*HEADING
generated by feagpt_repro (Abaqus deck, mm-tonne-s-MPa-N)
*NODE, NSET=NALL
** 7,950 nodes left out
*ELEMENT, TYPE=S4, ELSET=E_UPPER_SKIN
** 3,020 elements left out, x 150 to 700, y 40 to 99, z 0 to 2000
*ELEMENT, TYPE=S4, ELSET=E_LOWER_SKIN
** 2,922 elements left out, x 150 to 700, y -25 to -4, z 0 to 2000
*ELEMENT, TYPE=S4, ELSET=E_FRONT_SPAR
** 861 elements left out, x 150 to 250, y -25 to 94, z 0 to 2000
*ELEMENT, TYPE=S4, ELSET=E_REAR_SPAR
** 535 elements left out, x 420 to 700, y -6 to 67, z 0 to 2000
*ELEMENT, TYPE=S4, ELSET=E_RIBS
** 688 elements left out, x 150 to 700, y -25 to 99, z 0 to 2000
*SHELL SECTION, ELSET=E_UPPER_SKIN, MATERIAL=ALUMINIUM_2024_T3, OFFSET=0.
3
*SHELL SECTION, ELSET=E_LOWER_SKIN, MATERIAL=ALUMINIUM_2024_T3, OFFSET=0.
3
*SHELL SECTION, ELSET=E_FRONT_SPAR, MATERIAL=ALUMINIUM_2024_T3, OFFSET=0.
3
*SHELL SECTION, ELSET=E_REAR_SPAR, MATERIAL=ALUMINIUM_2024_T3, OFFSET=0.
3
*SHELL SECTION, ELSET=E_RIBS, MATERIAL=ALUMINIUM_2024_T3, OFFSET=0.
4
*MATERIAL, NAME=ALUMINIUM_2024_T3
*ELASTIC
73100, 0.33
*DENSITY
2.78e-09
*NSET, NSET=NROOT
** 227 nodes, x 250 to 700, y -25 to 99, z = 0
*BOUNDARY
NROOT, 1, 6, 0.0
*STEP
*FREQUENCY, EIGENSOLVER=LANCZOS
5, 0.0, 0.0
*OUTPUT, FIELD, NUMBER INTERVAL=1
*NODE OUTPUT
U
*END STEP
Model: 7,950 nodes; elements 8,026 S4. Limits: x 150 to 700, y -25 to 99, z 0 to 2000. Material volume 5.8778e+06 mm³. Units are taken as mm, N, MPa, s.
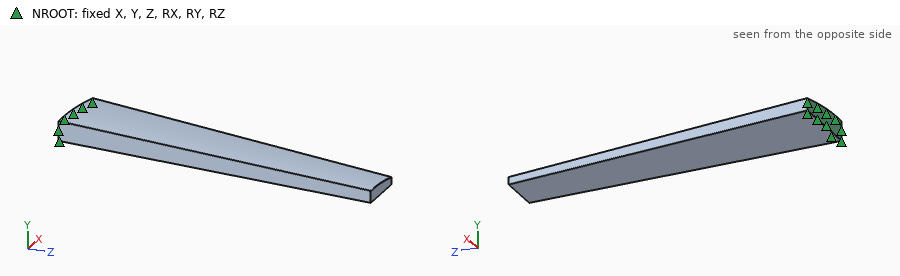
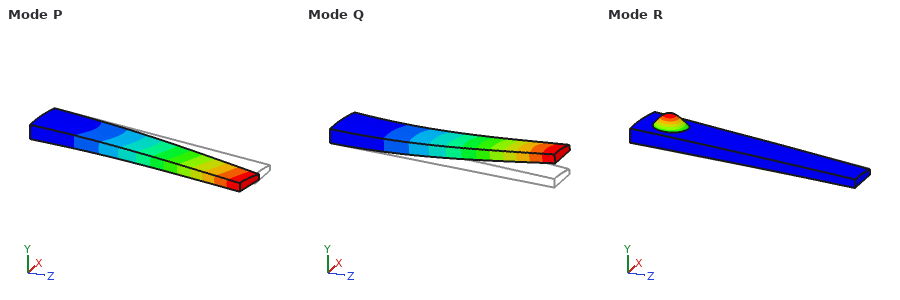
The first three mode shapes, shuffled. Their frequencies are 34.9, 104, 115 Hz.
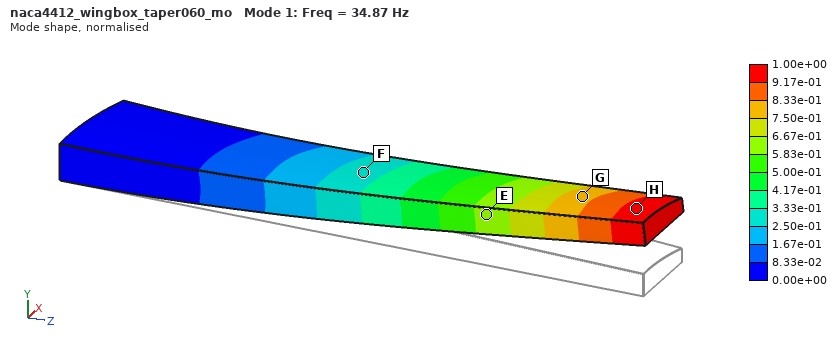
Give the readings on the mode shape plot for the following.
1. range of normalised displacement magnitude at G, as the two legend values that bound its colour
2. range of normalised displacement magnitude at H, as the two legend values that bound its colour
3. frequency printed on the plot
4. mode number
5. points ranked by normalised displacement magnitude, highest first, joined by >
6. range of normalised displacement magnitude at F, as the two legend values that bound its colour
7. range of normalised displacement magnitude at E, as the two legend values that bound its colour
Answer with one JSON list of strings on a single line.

["7.50e-01 to 8.33e-01", "9.17e-01 to 1.00e+00", "34.87 Hz", "1", "H > G > E > F", "2.50e-01 to 3.33e-01", "5.83e-01 to 6.67e-01"]
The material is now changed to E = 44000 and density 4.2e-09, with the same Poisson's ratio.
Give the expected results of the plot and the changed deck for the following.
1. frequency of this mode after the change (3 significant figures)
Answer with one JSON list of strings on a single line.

["22.0 Hz"]
